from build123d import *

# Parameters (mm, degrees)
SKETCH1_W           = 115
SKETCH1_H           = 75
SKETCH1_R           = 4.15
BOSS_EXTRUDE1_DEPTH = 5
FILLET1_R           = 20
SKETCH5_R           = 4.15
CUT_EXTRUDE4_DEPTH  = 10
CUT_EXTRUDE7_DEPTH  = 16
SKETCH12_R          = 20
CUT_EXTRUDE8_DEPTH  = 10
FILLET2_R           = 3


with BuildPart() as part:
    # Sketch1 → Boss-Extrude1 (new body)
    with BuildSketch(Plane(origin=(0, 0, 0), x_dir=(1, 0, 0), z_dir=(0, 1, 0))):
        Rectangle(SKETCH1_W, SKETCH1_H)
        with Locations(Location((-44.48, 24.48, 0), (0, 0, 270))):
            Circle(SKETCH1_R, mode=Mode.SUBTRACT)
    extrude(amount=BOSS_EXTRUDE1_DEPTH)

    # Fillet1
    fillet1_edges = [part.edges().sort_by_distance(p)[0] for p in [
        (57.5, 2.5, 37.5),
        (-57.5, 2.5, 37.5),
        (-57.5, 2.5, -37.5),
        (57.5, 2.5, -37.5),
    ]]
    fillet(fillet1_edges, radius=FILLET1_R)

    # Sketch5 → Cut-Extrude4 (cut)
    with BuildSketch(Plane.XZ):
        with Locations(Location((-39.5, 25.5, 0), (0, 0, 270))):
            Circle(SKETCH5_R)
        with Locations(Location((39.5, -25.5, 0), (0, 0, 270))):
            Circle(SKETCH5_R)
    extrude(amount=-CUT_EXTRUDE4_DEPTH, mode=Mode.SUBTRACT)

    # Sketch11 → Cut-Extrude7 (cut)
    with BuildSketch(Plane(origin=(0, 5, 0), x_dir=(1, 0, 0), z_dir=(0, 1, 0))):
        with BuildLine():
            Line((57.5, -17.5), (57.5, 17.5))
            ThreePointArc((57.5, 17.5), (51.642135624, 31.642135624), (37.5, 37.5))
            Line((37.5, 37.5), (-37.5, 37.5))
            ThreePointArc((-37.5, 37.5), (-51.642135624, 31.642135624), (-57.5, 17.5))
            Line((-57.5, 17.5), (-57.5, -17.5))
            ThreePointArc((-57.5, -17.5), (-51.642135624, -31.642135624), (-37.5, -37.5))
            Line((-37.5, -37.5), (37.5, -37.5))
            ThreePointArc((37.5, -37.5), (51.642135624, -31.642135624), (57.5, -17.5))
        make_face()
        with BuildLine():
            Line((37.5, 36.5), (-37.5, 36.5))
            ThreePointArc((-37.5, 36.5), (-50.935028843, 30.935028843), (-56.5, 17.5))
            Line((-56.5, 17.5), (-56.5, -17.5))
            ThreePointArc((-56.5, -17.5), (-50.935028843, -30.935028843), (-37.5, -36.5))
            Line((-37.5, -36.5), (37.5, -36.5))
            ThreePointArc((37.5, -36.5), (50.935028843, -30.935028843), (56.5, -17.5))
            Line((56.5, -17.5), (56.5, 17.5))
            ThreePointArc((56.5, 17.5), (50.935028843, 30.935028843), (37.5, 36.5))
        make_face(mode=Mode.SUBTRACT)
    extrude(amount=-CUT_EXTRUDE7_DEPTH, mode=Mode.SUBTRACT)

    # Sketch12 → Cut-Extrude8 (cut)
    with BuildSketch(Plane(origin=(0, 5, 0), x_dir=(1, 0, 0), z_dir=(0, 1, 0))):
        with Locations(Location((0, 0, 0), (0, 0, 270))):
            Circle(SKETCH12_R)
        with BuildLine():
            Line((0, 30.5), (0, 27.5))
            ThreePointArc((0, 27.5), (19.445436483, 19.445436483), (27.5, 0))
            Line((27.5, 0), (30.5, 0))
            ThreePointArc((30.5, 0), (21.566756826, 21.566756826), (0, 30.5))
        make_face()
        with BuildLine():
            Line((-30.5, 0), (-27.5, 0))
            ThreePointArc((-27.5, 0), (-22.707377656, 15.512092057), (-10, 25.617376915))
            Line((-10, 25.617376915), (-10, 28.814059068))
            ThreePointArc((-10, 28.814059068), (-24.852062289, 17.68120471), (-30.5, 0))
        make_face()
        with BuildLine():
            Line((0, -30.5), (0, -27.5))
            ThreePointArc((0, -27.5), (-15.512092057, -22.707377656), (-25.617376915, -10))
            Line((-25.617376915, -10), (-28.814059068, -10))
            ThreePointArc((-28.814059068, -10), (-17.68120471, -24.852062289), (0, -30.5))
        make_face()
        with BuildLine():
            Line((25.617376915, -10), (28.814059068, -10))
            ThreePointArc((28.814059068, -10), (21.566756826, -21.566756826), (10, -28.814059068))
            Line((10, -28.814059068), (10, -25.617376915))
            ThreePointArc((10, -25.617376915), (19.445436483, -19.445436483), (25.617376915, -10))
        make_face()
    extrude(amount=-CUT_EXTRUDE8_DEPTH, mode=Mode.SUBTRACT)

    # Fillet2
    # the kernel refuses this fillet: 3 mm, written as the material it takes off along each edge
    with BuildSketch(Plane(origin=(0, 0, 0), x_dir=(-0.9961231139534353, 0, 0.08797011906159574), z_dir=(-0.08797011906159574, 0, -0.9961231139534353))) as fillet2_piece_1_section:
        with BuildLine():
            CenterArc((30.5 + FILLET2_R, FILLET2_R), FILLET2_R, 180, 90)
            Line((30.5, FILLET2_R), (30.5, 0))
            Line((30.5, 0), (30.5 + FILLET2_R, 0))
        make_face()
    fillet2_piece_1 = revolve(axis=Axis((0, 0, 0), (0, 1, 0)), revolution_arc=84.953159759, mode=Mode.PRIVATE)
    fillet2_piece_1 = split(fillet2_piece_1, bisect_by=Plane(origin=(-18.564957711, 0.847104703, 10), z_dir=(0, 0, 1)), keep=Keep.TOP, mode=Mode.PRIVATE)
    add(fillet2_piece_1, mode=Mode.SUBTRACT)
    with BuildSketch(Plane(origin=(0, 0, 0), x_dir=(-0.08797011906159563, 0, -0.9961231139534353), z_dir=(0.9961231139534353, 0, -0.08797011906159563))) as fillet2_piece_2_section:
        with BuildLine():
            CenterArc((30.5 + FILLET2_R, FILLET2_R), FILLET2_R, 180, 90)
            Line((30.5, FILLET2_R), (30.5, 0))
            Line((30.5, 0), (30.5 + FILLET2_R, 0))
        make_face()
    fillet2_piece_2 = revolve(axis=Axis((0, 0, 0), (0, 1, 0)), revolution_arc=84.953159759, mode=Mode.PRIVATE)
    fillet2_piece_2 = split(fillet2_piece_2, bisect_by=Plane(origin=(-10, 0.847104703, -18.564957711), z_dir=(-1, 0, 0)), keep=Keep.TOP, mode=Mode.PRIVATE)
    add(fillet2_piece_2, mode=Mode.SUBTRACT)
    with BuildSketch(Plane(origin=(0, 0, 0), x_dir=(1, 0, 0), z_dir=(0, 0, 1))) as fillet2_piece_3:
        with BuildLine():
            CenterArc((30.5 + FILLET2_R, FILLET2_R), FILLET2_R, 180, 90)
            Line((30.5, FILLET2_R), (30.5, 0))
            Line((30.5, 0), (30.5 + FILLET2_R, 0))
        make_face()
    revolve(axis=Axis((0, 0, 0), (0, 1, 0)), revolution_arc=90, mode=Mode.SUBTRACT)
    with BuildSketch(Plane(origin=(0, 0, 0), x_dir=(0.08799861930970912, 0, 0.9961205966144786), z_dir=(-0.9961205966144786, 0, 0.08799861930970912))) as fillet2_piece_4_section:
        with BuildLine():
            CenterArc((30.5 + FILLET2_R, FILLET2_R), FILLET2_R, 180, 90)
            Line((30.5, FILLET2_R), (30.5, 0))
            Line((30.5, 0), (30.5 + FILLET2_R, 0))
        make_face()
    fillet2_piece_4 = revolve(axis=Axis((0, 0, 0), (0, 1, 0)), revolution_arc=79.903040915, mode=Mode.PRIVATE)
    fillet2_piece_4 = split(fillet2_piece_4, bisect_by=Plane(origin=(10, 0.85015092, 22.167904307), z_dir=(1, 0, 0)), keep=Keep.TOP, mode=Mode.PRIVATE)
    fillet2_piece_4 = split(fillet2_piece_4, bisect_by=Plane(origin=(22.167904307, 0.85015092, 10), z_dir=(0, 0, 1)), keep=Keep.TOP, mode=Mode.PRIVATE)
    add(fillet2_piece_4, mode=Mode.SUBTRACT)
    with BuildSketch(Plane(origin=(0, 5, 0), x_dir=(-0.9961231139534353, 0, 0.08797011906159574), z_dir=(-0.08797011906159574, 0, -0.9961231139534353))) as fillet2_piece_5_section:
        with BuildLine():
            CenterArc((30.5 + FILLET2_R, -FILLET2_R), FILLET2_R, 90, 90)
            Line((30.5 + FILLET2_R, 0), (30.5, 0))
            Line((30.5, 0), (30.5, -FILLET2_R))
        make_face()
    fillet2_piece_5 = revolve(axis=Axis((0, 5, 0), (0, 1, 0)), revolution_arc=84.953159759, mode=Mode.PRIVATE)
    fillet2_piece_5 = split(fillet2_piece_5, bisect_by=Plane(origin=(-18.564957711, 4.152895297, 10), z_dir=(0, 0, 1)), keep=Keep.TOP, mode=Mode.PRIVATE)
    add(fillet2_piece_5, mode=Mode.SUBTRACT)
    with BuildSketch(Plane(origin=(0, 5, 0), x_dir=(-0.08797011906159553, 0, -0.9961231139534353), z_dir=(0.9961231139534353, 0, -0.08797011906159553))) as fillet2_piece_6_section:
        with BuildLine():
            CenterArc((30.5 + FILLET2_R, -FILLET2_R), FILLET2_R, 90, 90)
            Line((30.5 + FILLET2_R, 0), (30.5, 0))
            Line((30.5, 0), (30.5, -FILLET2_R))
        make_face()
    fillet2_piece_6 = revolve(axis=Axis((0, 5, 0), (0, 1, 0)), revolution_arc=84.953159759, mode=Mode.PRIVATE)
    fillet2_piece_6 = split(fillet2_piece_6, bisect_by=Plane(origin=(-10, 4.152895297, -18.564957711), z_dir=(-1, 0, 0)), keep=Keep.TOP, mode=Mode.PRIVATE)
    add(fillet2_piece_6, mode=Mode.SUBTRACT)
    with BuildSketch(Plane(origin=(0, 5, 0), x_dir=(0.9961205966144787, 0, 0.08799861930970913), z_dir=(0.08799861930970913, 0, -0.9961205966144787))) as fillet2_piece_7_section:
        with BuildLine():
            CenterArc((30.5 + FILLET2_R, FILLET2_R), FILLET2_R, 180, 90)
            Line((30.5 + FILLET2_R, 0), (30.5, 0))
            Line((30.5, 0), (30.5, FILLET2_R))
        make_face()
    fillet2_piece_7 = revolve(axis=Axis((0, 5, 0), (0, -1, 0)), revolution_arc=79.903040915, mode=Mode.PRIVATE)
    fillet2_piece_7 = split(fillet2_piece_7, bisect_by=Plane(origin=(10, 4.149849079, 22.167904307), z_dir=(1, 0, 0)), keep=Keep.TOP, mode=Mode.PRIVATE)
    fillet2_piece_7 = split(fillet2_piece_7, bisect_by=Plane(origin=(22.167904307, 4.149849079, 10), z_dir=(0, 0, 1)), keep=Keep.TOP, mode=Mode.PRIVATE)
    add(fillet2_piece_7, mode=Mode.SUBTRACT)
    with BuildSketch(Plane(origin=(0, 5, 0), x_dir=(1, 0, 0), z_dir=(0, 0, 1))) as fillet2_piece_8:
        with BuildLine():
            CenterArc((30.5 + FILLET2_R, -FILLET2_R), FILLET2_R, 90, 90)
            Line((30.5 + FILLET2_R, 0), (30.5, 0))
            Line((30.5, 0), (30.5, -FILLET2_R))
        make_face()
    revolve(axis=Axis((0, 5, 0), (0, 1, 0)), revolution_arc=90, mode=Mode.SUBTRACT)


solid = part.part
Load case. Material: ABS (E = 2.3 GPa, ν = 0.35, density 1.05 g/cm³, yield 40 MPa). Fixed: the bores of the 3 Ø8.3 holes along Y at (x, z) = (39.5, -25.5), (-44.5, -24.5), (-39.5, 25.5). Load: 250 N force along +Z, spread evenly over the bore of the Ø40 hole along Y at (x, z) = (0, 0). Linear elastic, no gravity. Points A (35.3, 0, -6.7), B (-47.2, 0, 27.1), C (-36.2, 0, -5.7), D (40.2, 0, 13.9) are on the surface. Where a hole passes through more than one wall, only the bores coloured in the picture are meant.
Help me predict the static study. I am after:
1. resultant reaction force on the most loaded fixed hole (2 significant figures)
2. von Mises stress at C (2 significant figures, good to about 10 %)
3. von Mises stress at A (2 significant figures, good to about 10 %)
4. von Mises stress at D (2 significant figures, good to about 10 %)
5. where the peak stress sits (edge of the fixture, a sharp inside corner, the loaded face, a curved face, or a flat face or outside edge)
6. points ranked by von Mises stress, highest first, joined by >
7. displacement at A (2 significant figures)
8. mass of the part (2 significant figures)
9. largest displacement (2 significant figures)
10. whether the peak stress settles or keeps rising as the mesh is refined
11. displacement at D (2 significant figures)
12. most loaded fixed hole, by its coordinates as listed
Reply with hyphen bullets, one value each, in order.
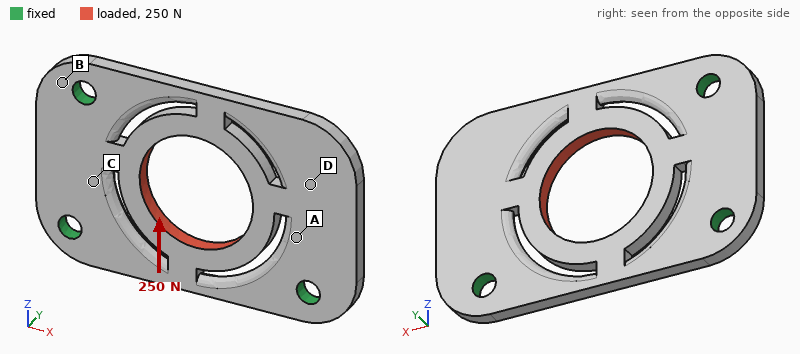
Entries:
- 120 N
- 1.3 MPa
- 1.8 MPa
- 0.76 MPa
- a sharp inside corner
- A > C > D > B
- 12 µm
- 31 g
- 61 µm
- keeps rising
- 15 µm
- (39.5, -25.5)
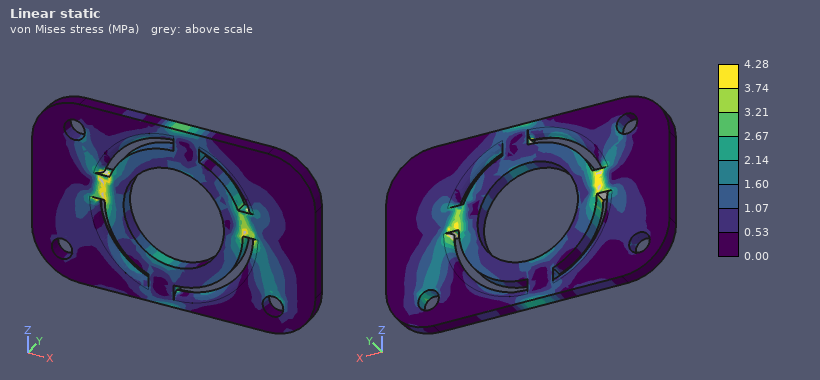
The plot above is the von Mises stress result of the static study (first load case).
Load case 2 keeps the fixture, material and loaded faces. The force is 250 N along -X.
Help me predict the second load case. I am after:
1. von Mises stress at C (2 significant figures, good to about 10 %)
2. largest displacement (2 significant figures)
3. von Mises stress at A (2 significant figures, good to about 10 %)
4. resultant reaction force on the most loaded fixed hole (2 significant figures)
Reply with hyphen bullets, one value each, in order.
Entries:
- 0.83 MPa
- 76 µm
- 0.99 MPa
- 87 N
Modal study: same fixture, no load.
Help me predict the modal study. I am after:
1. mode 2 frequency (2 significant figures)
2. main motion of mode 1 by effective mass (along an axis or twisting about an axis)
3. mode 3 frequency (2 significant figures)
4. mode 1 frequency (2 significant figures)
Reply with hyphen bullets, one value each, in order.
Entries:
- 990 Hz
- along Y
- 1100 Hz
- 410 Hz
